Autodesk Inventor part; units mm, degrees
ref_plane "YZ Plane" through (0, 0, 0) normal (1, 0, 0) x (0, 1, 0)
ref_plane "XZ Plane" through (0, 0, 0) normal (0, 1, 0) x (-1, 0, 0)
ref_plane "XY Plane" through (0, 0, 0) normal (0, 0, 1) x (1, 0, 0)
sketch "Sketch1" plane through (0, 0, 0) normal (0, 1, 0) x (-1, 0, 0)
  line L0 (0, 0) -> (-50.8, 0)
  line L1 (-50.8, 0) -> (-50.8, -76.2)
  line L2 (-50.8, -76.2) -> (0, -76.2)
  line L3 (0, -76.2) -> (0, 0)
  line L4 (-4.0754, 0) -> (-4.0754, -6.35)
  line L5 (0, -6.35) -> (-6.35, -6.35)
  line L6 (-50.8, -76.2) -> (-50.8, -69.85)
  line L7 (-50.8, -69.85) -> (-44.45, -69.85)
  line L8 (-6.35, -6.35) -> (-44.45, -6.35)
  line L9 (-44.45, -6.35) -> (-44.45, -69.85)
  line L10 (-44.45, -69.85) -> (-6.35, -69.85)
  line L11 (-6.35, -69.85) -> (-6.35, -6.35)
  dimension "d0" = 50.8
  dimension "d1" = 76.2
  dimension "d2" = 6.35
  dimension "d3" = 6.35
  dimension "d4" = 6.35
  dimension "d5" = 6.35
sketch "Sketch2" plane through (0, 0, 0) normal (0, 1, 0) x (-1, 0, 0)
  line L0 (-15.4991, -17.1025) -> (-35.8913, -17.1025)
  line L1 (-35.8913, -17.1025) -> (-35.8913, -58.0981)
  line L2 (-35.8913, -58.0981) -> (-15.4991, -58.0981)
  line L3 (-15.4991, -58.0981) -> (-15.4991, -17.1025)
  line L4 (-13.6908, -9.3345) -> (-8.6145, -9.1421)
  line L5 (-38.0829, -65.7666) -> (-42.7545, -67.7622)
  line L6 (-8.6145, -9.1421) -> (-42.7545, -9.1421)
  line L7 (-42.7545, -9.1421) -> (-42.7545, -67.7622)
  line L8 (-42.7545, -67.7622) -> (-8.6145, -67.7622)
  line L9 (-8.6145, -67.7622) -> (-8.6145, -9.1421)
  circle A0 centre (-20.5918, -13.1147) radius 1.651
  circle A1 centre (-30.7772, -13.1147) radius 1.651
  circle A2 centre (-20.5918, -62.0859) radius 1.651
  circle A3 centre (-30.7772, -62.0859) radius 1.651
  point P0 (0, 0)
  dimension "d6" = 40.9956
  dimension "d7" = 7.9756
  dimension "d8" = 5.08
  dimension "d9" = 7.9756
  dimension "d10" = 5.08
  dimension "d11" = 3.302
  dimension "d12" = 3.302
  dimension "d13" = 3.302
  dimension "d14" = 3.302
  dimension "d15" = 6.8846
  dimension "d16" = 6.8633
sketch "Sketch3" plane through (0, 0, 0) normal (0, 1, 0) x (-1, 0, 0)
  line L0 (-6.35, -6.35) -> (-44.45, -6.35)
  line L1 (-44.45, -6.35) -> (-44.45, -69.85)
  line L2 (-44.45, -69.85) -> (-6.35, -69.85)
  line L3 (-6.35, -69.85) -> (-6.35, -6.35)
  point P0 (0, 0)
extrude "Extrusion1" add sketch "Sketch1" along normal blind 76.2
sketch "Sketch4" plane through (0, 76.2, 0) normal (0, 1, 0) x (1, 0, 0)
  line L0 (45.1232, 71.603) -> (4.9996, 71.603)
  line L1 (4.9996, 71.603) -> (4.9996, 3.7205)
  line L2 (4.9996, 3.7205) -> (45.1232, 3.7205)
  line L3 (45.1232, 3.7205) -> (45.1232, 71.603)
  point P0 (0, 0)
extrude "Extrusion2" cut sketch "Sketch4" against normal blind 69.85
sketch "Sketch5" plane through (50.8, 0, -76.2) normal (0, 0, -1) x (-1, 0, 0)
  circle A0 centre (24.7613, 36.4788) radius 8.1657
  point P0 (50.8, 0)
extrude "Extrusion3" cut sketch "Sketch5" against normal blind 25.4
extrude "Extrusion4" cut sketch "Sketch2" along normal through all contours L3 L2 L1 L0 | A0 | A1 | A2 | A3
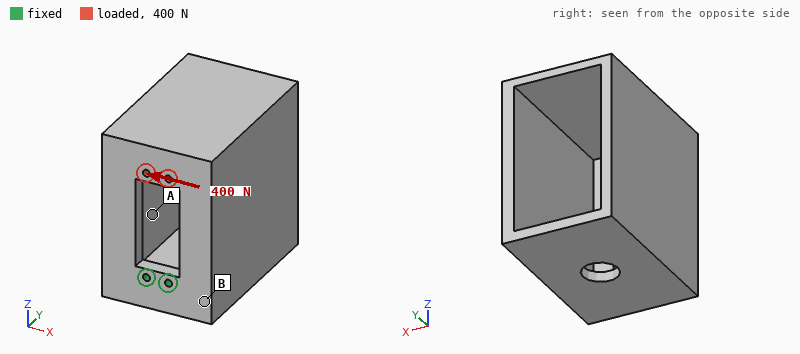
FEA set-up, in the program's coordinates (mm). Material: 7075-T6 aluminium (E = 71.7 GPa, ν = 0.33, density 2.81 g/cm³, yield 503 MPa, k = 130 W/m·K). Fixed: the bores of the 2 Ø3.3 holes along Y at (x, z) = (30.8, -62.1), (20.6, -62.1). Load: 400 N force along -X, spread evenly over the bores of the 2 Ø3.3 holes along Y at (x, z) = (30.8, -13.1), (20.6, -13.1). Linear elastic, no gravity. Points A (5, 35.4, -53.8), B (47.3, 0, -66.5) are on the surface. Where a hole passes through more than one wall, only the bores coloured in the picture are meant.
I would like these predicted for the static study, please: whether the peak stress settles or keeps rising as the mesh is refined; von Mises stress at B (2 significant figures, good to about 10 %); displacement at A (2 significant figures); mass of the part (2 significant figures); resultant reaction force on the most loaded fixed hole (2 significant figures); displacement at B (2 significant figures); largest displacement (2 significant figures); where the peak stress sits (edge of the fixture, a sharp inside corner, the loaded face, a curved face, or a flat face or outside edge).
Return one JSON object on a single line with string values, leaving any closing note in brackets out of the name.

{"whether the peak stress settles or keeps rising as the mesh is refined": "keeps rising", "von Mises stress at B": "8.7 MPa", "displacement at A": "24 µm", "mass of the part": "280 g", "resultant reaction force on the most loaded fixed hole": "1.4 kN", "displacement at B": "16 µm", "largest displacement": "78 µm", "where the peak stress sits": "edge of the fixture"}
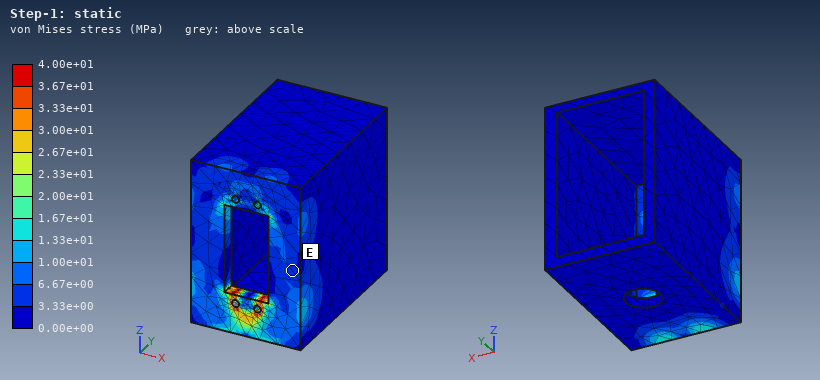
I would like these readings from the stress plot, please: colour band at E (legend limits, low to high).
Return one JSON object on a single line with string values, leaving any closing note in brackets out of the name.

{"colour band at E": "3.33e+00 to 6.67e+00 MPa"}
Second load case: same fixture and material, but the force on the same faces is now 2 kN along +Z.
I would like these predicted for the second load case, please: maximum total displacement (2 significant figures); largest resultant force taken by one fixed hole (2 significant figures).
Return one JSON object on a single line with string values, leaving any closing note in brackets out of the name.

{"maximum total displacement": "23 µm", "largest resultant force taken by one fixed hole": "1.2 kN"}
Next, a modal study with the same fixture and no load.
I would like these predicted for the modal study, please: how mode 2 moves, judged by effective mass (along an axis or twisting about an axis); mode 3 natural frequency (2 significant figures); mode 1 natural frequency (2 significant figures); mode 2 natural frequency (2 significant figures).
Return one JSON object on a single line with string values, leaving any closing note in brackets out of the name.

{"how mode 2 moves, judged by effective mass": "along X", "mode 3 natural frequency": "1400 Hz", "mode 1 natural frequency": "430 Hz", "mode 2 natural frequency": "740 Hz"}
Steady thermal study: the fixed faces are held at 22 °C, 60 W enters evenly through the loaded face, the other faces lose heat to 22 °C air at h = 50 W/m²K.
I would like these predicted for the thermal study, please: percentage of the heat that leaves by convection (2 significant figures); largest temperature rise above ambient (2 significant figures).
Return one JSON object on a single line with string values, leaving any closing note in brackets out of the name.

{"percentage of the heat that leaves by convection": "63 %", "largest temperature rise above ambient": "67 K"}
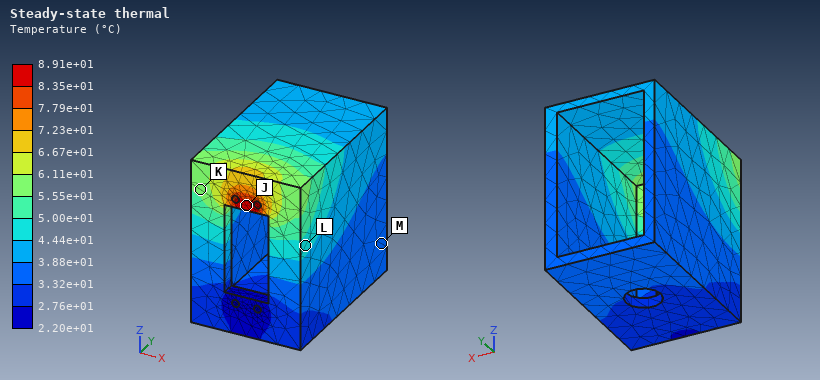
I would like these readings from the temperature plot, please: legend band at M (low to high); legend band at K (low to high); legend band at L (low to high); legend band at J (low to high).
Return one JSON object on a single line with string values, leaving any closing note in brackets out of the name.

{"legend band at M": "3.32e+01 to 3.88e+01 °C", "legend band at K": "5.55e+01 to 6.11e+01 °C", "legend band at L": "4.44e+01 to 5.00e+01 °C", "legend band at J": "8.35e+01 to 8.91e+01 °C"}
